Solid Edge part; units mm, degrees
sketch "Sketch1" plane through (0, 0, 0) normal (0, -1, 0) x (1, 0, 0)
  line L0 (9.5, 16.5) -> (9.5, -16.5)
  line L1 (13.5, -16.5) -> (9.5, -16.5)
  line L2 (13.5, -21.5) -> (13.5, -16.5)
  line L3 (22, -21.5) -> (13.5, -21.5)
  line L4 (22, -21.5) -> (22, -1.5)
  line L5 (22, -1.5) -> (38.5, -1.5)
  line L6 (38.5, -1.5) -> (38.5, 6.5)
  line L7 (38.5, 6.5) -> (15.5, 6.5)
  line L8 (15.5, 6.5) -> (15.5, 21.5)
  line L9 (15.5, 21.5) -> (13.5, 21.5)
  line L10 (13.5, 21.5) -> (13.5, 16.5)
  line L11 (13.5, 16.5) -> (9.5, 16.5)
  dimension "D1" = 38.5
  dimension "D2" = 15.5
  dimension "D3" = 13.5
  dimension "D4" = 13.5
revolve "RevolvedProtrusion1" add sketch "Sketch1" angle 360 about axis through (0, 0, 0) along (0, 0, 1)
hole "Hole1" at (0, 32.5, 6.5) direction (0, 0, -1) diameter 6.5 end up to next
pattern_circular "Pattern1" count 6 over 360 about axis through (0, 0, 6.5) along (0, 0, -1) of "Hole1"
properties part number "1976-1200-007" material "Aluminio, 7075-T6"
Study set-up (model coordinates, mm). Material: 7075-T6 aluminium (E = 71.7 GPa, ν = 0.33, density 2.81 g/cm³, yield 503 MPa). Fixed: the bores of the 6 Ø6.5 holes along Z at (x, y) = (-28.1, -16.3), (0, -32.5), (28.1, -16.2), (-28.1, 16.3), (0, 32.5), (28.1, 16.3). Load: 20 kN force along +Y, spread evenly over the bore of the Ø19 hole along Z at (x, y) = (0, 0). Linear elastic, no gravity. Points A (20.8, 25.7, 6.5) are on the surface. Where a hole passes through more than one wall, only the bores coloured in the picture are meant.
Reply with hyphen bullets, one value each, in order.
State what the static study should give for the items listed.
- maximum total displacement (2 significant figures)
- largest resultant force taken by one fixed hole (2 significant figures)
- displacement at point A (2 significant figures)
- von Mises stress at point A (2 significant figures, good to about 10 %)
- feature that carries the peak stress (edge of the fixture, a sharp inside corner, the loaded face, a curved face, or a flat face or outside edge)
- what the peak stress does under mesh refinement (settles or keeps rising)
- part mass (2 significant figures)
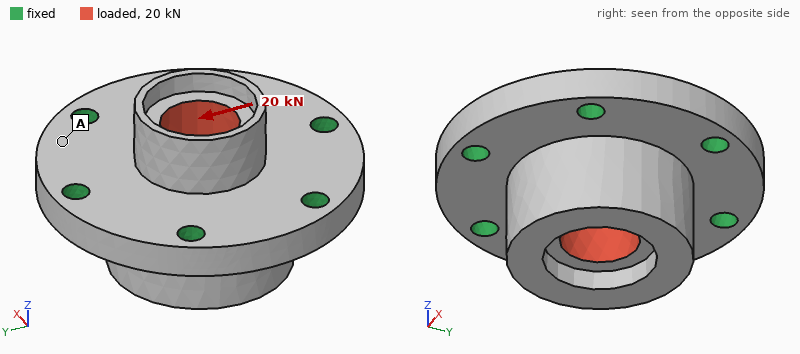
- 15 µm
- 4.9 kN
- 3.9 µm
- 11 MPa
- edge of the fixture
- keeps rising
- 180 g
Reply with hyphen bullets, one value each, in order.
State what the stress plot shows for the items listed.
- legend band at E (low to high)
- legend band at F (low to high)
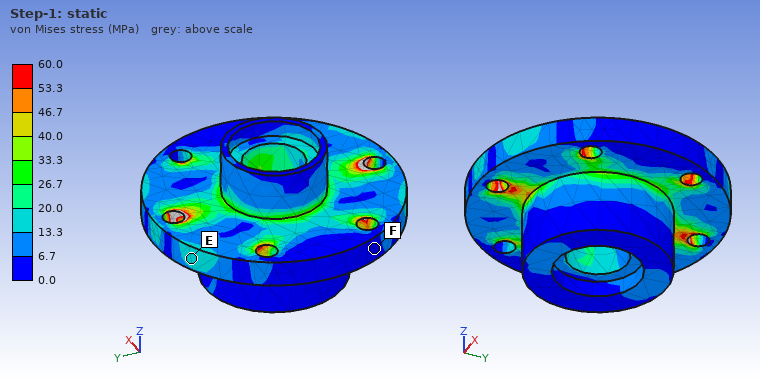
- 13.3 to 20.0 MPa
- 0.0 to 6.7 MPa
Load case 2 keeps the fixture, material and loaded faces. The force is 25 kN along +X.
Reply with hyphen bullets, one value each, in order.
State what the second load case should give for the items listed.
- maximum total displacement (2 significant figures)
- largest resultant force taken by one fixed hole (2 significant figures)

- 19 µm
- 5.4 kN
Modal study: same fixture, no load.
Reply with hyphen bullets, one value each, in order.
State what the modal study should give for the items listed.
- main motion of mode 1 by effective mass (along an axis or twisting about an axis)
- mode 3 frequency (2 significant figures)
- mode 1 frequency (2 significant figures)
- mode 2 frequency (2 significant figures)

- along Z
- 16 kHz
- 14 kHz
- 15 kHz
